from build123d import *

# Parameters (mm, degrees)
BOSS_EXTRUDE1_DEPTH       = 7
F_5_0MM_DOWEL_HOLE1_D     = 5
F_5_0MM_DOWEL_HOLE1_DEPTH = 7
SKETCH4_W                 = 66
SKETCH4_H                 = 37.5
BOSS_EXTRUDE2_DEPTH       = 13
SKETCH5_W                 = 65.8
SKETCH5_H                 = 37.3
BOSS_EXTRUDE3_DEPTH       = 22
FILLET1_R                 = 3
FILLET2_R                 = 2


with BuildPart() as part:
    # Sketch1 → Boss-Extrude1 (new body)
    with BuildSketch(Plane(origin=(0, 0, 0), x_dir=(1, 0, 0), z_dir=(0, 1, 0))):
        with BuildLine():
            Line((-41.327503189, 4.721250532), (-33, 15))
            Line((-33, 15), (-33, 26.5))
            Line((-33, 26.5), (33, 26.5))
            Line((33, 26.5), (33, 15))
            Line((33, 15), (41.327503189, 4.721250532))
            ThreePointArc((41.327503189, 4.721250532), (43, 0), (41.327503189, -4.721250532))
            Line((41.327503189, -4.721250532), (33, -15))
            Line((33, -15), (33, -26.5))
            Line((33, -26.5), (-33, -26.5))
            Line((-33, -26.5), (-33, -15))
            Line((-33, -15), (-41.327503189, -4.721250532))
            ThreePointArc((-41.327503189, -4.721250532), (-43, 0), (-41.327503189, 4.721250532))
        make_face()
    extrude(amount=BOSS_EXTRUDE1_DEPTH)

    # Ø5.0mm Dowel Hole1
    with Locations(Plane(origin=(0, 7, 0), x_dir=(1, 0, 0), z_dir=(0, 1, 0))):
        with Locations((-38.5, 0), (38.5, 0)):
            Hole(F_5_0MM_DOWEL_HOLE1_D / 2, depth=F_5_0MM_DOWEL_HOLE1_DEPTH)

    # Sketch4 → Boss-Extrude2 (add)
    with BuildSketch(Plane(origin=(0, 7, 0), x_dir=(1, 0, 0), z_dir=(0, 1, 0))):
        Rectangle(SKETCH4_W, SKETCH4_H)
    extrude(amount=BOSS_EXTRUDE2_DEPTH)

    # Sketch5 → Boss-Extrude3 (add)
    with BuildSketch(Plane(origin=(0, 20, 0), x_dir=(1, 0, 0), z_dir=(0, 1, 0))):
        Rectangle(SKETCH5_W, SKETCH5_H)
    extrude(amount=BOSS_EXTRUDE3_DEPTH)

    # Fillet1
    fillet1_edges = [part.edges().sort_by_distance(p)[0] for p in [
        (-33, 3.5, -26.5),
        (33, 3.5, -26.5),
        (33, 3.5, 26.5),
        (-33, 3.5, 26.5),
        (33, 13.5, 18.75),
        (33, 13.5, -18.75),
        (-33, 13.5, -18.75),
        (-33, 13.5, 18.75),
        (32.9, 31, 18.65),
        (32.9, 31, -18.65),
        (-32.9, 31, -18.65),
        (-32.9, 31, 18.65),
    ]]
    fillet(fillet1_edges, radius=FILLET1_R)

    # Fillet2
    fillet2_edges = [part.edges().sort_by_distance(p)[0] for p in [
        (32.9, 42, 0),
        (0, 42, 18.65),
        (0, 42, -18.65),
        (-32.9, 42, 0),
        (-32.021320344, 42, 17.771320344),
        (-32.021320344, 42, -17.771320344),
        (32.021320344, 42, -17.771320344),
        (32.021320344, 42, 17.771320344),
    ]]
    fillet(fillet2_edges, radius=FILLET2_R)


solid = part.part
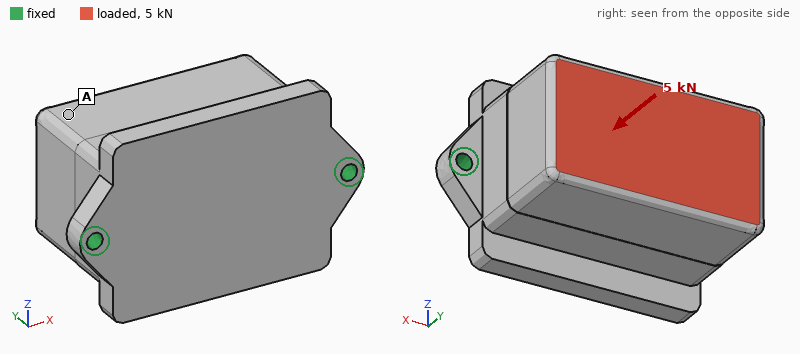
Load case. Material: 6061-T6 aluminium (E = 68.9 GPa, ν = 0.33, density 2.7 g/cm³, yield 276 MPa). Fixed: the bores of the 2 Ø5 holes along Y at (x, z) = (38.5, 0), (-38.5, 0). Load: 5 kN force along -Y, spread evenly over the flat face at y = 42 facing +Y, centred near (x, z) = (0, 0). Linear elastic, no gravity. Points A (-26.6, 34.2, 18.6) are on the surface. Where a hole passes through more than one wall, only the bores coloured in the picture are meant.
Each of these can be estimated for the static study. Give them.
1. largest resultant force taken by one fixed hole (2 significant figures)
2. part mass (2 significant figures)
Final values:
2.7 kN
300 g
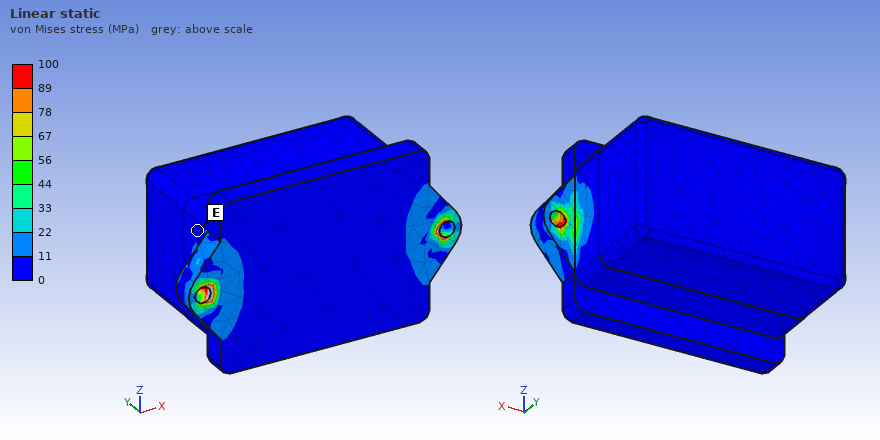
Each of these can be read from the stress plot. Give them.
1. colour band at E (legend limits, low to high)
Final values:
0 to 11 MPa
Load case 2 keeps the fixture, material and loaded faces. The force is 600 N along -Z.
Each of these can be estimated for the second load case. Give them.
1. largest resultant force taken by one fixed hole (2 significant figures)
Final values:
300 N
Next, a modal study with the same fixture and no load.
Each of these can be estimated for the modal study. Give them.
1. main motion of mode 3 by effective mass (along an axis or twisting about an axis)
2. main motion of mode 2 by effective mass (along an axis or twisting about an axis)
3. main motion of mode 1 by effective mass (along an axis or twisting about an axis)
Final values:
along X
along Y
along Z
